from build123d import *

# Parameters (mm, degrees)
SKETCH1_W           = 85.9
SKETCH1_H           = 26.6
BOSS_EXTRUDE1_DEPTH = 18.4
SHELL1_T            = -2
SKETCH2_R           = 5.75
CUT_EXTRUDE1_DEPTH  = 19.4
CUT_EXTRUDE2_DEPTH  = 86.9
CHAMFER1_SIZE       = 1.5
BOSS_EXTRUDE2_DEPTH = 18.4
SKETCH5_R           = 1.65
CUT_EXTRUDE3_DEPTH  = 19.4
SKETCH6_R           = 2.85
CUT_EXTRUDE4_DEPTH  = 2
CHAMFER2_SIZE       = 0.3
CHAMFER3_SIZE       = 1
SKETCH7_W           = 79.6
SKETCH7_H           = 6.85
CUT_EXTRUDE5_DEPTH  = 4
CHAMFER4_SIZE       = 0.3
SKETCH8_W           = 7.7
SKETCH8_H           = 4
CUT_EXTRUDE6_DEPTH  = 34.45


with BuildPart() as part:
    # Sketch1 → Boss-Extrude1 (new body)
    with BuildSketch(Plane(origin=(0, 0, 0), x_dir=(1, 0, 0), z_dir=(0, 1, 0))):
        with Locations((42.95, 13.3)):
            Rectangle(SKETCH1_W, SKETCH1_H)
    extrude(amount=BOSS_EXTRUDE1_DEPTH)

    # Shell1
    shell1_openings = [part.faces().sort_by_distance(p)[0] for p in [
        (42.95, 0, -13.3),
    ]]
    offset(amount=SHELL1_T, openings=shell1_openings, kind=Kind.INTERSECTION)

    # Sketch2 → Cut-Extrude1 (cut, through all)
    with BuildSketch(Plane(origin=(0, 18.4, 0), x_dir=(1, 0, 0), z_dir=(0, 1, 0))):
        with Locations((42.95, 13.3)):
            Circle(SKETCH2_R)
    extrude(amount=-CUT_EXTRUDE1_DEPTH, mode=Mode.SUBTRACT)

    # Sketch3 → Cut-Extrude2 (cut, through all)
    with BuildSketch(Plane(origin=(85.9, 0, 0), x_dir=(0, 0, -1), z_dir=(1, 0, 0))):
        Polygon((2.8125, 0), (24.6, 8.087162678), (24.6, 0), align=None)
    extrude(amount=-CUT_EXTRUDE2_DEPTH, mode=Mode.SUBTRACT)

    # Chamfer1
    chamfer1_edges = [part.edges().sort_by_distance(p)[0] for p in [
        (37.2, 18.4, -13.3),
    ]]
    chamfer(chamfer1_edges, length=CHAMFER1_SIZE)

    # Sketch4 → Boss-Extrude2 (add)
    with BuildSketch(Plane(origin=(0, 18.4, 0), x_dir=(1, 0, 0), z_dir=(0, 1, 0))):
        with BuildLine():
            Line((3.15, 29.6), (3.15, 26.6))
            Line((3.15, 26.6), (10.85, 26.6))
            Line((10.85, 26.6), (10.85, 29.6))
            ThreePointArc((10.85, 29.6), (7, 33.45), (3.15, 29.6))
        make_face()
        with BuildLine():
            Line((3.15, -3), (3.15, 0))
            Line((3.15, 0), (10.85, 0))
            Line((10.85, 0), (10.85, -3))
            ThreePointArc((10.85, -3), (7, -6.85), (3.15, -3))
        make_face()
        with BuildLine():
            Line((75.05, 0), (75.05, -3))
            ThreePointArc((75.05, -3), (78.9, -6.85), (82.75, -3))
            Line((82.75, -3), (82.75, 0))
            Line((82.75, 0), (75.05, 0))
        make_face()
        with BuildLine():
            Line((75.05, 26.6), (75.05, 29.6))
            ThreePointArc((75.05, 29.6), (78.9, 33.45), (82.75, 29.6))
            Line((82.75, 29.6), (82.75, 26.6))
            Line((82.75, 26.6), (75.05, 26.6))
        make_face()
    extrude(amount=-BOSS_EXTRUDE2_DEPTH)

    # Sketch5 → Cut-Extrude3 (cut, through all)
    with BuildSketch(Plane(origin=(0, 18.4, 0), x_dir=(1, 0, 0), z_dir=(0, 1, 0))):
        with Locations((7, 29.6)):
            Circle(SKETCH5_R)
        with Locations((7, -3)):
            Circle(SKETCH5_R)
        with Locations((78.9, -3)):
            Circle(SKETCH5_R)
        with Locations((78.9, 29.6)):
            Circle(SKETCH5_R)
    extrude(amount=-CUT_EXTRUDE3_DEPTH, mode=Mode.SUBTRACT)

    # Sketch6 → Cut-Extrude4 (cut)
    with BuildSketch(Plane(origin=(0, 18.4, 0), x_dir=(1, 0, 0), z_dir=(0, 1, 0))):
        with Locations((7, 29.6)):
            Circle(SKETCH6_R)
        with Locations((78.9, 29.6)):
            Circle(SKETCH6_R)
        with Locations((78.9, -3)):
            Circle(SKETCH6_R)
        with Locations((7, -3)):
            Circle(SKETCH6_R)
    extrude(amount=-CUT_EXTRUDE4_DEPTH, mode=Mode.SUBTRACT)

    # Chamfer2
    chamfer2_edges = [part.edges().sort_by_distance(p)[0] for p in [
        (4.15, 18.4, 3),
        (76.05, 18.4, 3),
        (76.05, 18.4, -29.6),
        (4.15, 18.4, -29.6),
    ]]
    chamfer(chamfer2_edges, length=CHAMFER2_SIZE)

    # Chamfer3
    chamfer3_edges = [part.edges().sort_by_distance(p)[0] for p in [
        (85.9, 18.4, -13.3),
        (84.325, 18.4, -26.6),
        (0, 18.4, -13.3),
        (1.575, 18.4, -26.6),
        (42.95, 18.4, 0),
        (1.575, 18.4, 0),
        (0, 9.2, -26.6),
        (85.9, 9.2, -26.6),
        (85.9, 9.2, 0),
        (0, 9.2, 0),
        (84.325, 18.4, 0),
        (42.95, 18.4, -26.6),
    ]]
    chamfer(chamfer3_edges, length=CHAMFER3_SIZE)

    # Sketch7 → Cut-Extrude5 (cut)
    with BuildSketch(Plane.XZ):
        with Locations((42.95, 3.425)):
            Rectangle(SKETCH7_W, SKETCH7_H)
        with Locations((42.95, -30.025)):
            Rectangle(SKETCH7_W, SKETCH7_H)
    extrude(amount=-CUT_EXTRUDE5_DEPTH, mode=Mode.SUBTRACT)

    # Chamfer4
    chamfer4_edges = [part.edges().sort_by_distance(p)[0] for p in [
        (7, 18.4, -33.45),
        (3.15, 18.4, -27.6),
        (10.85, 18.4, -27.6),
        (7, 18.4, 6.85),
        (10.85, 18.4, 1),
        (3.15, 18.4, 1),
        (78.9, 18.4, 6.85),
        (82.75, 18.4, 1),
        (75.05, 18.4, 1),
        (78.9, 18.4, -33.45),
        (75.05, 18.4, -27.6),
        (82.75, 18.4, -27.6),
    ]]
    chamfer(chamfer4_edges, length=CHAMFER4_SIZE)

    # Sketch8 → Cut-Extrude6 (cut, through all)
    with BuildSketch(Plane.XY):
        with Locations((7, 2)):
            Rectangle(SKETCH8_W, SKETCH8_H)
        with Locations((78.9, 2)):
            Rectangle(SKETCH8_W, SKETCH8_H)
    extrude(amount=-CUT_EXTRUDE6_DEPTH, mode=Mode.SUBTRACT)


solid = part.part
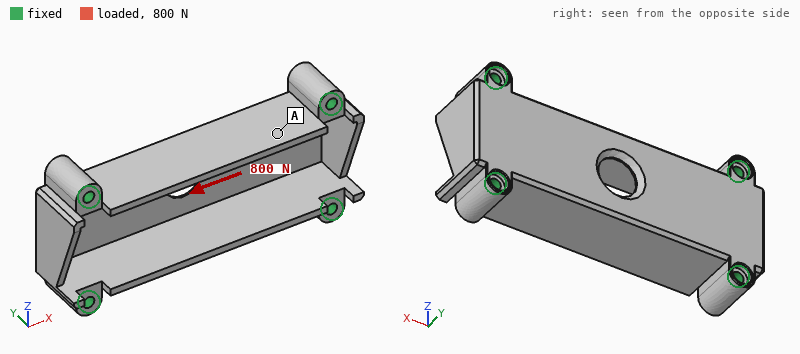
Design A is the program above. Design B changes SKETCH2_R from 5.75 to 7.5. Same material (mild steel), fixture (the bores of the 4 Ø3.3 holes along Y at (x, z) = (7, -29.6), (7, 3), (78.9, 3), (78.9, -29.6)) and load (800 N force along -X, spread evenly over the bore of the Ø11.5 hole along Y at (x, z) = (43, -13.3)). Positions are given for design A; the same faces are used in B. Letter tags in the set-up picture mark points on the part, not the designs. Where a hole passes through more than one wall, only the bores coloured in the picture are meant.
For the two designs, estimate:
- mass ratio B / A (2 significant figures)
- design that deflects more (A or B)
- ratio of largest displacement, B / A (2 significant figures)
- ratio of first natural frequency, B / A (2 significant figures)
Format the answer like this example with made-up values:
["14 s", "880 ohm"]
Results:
["0.99", "A", "0.92", "0.98"]
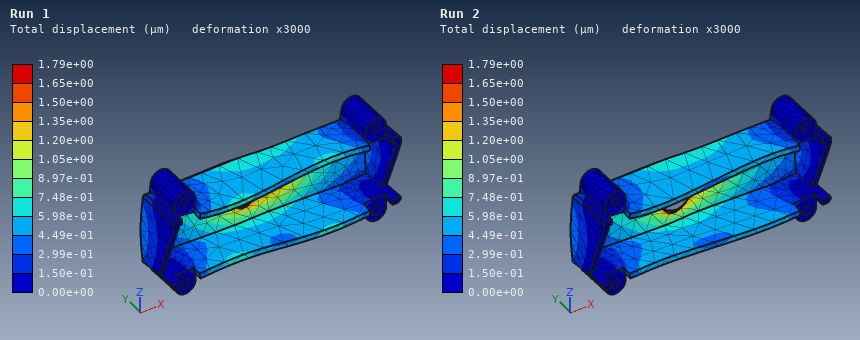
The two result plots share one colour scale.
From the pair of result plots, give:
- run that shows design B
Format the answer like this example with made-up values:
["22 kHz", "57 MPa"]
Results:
["Run 2"]
